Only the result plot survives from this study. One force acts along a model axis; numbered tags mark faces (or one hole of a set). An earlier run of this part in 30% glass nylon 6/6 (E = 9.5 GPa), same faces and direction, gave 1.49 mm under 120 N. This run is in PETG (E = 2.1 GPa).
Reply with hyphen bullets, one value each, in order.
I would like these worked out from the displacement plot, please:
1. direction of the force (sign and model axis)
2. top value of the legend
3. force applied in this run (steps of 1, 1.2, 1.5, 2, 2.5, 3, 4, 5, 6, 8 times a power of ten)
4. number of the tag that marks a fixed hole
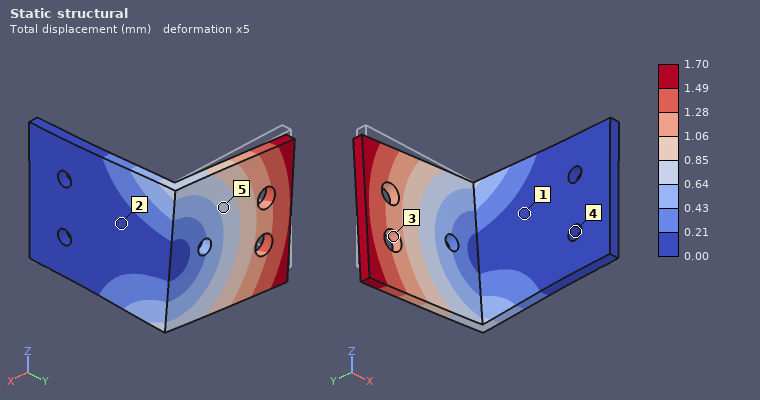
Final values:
- -Z
- 1.70 mm
- 30 N
- 4
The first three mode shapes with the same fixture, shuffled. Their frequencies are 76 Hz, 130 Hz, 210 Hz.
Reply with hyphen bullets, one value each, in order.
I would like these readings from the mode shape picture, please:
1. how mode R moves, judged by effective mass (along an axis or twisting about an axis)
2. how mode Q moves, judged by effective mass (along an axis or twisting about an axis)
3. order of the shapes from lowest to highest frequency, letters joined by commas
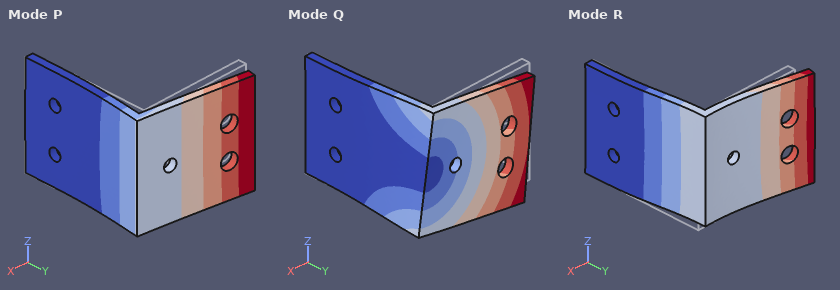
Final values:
- along X
- along Z
- P, Q, R
